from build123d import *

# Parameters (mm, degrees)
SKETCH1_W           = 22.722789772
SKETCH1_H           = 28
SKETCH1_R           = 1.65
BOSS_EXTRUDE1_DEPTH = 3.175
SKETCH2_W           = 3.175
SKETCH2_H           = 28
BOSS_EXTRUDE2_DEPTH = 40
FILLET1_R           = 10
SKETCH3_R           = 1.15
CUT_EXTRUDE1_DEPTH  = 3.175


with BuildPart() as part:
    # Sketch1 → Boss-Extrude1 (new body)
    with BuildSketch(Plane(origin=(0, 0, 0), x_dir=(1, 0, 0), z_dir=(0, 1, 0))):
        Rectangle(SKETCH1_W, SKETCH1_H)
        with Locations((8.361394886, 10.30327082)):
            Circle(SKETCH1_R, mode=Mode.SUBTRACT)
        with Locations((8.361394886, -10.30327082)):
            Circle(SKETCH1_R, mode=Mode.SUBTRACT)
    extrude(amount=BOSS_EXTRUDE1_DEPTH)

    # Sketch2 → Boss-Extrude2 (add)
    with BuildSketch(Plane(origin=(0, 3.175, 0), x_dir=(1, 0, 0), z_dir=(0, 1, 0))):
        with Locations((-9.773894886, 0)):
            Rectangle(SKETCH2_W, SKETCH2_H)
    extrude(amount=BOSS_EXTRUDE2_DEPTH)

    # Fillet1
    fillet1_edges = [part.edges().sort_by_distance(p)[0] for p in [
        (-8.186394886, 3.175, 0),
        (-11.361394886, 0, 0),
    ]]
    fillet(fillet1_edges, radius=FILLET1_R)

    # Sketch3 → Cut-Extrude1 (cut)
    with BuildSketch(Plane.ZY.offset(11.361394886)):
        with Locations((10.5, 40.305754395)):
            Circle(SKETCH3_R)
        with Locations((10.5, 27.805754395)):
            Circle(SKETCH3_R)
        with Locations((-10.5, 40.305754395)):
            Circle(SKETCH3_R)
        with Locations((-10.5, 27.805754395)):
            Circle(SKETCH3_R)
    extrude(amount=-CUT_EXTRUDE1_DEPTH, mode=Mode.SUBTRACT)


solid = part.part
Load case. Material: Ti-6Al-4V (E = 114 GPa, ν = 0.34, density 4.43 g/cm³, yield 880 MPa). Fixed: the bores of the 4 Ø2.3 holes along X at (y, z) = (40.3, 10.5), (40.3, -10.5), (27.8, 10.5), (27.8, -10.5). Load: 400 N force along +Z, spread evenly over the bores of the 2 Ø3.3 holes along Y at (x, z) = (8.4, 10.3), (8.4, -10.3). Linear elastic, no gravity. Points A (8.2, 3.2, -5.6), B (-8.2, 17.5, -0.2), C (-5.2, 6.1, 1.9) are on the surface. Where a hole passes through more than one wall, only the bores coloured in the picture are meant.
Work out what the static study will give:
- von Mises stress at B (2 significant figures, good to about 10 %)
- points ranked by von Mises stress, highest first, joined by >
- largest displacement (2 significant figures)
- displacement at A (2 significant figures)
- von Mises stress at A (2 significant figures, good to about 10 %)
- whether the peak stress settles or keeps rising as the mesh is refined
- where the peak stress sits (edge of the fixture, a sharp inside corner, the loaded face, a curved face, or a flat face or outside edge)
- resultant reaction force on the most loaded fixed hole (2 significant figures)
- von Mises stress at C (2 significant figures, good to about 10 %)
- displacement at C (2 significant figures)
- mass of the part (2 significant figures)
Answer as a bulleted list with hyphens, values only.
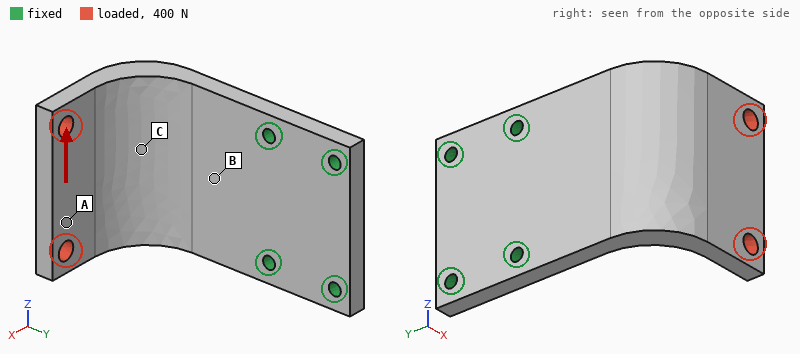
- 92 MPa
- B > C > A
- 0.18 mm
- 0.13 mm
- 16 MPa
- keeps rising
- edge of the fixture
- 600 N
- 68 MPa
- 0.034 mm
- 24 g
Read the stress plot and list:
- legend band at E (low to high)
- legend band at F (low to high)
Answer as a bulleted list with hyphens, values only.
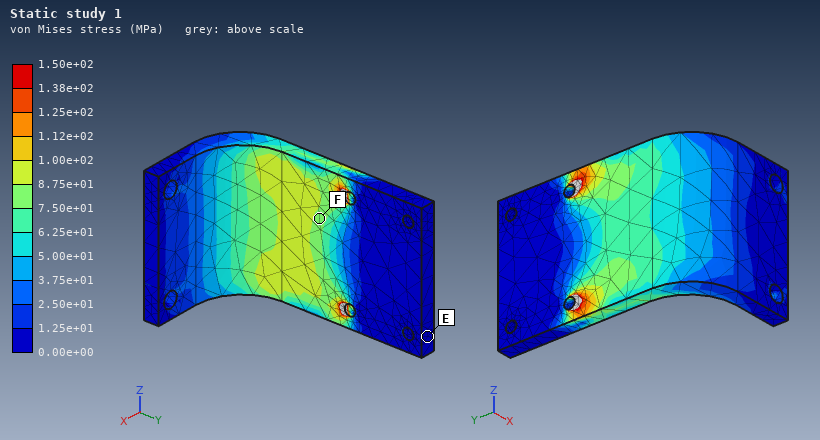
- 0.00e+00 to 1.25e+01 MPa
- 7.50e+01 to 8.75e+01 MPa
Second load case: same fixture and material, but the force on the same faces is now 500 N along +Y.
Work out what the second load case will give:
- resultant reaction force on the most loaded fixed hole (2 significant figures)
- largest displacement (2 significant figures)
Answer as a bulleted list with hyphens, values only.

- 250 N
- 0.63 mm
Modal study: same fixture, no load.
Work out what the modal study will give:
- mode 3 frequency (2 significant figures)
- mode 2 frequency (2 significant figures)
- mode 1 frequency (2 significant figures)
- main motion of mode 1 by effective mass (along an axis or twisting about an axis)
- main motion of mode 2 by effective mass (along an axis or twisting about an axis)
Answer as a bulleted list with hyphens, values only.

- 6900 Hz
- 3700 Hz
- 1600 Hz
- along X
- along Z
